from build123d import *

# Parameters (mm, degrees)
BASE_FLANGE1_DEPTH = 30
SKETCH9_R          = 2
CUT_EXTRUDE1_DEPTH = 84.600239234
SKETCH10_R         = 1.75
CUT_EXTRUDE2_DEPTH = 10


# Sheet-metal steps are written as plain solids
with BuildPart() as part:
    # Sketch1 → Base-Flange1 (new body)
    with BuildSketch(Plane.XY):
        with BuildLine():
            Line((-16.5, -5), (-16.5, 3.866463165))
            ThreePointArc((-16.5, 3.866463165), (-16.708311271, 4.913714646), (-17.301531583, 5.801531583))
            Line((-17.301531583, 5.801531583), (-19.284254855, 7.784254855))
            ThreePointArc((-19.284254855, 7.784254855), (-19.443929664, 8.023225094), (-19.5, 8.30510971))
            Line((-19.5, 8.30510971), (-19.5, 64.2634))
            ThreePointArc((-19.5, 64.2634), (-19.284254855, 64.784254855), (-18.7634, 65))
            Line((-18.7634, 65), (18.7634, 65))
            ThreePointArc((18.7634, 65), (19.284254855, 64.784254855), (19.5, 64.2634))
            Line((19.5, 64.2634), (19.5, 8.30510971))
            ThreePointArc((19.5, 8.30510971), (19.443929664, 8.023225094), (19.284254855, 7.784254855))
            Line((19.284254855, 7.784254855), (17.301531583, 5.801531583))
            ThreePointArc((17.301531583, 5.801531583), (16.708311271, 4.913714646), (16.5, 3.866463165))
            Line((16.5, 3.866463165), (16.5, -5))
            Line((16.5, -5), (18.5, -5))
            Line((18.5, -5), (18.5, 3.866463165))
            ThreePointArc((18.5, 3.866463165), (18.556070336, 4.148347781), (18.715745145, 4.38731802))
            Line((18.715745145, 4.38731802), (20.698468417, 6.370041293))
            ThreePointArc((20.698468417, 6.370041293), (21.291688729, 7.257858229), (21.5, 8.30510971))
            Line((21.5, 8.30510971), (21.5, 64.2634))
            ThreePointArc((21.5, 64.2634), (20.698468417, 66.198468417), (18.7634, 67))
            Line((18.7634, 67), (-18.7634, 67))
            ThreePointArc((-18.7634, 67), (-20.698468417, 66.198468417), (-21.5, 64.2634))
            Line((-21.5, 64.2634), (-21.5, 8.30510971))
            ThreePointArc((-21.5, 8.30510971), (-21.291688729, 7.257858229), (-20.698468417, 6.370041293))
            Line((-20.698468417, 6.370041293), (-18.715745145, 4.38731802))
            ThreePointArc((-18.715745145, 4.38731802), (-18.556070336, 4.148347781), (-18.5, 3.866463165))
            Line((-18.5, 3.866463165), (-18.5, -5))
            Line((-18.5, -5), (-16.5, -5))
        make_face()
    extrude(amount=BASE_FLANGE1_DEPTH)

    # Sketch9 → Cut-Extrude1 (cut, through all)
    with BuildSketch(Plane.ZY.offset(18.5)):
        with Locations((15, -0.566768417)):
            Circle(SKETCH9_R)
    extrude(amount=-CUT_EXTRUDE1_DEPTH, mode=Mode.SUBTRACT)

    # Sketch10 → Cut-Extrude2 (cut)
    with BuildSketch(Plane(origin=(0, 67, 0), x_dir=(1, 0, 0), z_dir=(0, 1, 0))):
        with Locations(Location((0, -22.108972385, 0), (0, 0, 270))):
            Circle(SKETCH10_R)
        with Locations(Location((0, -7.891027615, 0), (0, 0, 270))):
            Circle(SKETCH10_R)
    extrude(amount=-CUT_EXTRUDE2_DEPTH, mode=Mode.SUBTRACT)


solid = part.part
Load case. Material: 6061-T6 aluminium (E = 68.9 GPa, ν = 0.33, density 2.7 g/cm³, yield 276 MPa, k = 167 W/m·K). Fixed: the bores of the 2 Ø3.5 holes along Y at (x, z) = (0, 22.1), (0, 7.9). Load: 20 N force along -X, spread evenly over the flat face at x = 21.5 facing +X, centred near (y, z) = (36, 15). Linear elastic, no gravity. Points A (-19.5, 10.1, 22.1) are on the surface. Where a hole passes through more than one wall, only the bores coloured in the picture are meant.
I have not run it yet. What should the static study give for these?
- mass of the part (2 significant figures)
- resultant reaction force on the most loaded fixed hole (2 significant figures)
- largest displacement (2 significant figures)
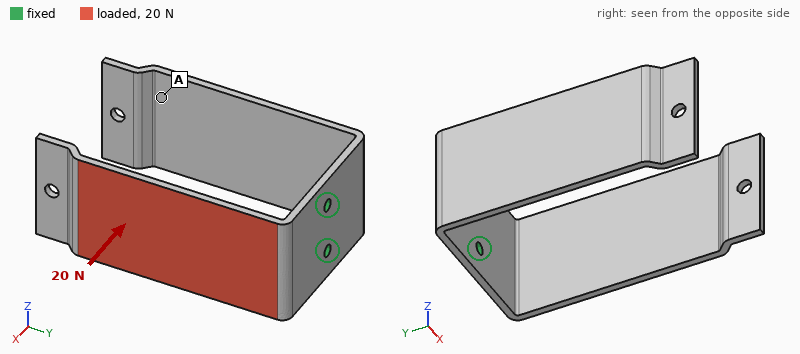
30 g
11 N
0.99 mm
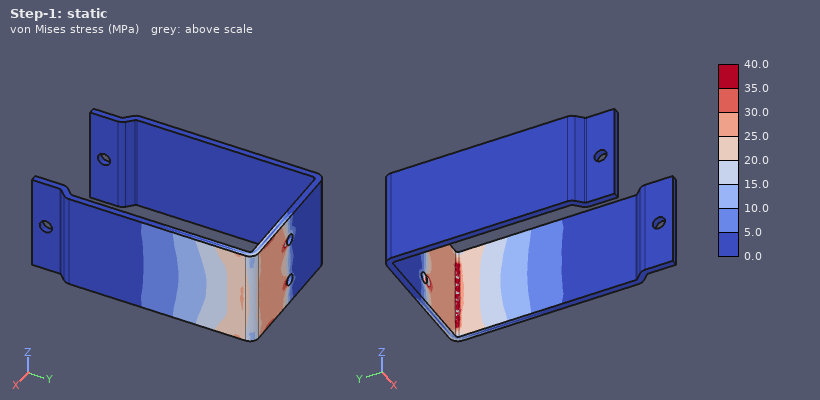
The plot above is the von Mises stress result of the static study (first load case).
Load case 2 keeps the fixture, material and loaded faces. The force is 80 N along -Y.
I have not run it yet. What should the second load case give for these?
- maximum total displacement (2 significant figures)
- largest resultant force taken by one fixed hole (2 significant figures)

0.93 mm
40 N
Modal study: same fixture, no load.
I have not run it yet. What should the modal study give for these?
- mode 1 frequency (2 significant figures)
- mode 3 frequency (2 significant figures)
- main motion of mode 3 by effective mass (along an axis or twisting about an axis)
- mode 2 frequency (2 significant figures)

230 Hz
460 Hz
twisting about Y
230 Hz
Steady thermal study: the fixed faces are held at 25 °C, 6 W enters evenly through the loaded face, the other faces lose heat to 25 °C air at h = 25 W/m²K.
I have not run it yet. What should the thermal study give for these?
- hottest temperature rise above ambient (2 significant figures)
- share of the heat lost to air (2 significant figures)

21 K
26 %
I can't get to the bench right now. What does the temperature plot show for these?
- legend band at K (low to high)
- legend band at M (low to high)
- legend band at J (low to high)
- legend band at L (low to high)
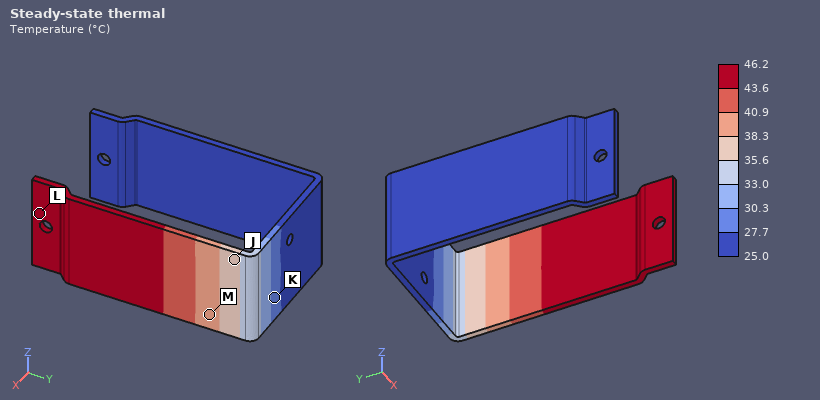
27.7 to 30.3 °C
38.3 to 40.9 °C
35.6 to 38.3 °C
43.6 to 46.2 °C
